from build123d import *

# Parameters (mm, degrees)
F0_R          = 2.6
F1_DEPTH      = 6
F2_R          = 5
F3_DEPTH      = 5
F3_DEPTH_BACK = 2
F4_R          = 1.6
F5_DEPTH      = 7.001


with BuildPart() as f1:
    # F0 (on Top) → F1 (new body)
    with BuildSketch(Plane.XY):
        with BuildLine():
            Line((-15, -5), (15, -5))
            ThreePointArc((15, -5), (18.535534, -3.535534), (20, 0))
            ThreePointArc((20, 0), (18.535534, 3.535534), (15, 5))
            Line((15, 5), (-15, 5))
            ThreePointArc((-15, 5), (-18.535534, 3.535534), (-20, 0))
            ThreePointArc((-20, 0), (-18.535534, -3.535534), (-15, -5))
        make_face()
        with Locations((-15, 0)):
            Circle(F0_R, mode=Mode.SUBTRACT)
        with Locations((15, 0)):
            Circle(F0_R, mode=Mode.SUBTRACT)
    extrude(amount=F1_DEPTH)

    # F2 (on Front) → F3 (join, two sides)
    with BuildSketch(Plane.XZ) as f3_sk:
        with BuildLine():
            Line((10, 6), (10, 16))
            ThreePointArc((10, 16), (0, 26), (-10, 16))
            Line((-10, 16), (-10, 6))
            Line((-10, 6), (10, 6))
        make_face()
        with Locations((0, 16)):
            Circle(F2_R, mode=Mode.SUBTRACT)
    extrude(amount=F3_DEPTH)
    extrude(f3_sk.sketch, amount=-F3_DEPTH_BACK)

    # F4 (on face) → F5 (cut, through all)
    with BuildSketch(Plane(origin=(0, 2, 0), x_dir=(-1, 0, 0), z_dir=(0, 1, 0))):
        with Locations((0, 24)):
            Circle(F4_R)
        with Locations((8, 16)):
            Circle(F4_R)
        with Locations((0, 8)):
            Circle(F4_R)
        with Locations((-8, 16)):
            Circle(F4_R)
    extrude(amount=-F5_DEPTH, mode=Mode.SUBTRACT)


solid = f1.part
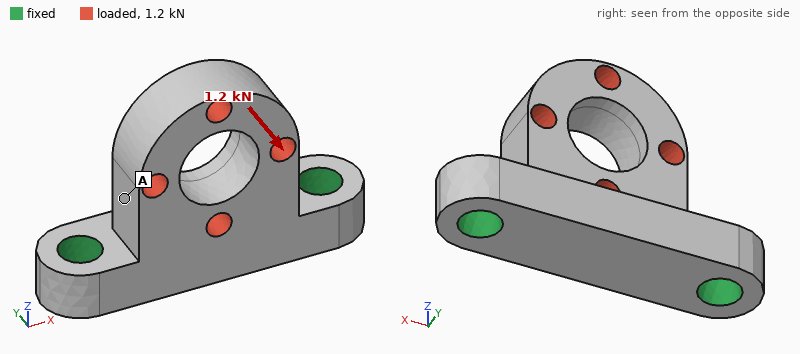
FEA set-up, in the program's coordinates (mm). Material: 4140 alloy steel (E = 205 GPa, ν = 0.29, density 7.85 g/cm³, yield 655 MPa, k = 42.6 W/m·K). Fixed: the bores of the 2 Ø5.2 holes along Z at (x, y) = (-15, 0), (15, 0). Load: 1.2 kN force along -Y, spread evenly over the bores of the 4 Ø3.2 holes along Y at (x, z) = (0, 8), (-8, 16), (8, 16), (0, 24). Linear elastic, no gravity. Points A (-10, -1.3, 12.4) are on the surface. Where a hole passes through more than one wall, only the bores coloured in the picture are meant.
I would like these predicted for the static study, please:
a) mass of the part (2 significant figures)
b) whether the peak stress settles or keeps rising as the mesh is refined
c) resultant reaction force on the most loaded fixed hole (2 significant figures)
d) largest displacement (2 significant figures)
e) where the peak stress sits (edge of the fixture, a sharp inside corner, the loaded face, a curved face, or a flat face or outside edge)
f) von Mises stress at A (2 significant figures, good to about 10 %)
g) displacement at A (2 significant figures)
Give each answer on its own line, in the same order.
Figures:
29 g
keeps rising
600 N
52 µm
edge of the fixture
27 MPa
15 µm
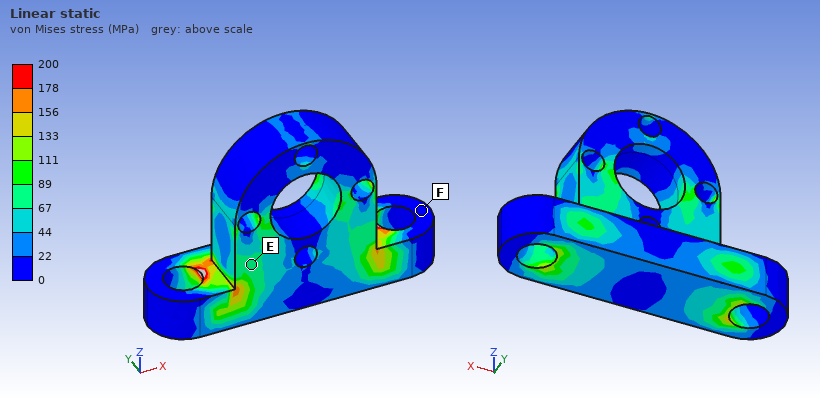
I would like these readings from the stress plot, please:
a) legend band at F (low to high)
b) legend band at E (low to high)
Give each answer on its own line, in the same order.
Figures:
0 to 22 MPa
67 to 89 MPa
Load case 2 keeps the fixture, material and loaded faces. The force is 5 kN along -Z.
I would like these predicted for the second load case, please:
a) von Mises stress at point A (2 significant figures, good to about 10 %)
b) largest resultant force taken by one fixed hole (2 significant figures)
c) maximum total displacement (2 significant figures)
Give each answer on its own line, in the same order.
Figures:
69 MPa
2.6 kN
18 µm
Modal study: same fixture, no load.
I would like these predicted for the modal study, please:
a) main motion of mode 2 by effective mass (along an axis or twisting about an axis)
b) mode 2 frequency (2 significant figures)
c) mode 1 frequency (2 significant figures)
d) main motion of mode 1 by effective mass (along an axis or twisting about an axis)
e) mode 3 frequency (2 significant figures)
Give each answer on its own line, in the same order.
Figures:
along X
17 kHz
8900 Hz
along Y
22 kHz
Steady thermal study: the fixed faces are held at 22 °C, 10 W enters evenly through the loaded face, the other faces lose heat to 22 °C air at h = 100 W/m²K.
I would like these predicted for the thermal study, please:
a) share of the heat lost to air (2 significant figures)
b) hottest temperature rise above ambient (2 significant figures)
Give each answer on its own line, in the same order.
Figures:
30 %
37 K
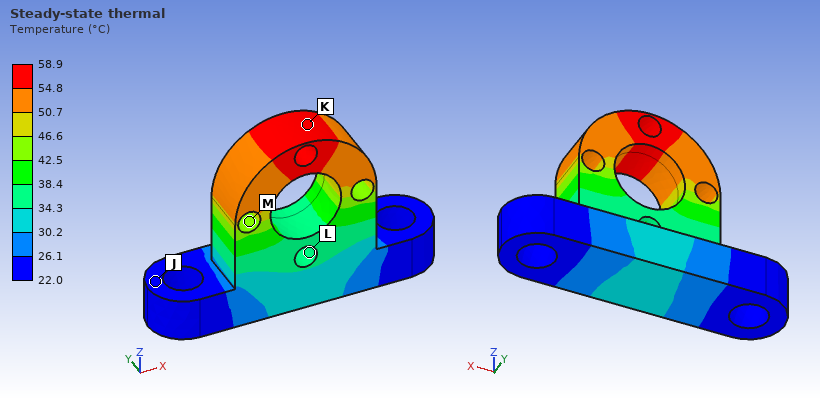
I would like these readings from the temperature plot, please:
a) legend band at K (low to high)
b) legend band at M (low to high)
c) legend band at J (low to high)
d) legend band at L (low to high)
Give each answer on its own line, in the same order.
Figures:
54.8 to 58.9 °C
42.5 to 46.6 °C
22.0 to 26.1 °C
34.3 to 38.4 °C
